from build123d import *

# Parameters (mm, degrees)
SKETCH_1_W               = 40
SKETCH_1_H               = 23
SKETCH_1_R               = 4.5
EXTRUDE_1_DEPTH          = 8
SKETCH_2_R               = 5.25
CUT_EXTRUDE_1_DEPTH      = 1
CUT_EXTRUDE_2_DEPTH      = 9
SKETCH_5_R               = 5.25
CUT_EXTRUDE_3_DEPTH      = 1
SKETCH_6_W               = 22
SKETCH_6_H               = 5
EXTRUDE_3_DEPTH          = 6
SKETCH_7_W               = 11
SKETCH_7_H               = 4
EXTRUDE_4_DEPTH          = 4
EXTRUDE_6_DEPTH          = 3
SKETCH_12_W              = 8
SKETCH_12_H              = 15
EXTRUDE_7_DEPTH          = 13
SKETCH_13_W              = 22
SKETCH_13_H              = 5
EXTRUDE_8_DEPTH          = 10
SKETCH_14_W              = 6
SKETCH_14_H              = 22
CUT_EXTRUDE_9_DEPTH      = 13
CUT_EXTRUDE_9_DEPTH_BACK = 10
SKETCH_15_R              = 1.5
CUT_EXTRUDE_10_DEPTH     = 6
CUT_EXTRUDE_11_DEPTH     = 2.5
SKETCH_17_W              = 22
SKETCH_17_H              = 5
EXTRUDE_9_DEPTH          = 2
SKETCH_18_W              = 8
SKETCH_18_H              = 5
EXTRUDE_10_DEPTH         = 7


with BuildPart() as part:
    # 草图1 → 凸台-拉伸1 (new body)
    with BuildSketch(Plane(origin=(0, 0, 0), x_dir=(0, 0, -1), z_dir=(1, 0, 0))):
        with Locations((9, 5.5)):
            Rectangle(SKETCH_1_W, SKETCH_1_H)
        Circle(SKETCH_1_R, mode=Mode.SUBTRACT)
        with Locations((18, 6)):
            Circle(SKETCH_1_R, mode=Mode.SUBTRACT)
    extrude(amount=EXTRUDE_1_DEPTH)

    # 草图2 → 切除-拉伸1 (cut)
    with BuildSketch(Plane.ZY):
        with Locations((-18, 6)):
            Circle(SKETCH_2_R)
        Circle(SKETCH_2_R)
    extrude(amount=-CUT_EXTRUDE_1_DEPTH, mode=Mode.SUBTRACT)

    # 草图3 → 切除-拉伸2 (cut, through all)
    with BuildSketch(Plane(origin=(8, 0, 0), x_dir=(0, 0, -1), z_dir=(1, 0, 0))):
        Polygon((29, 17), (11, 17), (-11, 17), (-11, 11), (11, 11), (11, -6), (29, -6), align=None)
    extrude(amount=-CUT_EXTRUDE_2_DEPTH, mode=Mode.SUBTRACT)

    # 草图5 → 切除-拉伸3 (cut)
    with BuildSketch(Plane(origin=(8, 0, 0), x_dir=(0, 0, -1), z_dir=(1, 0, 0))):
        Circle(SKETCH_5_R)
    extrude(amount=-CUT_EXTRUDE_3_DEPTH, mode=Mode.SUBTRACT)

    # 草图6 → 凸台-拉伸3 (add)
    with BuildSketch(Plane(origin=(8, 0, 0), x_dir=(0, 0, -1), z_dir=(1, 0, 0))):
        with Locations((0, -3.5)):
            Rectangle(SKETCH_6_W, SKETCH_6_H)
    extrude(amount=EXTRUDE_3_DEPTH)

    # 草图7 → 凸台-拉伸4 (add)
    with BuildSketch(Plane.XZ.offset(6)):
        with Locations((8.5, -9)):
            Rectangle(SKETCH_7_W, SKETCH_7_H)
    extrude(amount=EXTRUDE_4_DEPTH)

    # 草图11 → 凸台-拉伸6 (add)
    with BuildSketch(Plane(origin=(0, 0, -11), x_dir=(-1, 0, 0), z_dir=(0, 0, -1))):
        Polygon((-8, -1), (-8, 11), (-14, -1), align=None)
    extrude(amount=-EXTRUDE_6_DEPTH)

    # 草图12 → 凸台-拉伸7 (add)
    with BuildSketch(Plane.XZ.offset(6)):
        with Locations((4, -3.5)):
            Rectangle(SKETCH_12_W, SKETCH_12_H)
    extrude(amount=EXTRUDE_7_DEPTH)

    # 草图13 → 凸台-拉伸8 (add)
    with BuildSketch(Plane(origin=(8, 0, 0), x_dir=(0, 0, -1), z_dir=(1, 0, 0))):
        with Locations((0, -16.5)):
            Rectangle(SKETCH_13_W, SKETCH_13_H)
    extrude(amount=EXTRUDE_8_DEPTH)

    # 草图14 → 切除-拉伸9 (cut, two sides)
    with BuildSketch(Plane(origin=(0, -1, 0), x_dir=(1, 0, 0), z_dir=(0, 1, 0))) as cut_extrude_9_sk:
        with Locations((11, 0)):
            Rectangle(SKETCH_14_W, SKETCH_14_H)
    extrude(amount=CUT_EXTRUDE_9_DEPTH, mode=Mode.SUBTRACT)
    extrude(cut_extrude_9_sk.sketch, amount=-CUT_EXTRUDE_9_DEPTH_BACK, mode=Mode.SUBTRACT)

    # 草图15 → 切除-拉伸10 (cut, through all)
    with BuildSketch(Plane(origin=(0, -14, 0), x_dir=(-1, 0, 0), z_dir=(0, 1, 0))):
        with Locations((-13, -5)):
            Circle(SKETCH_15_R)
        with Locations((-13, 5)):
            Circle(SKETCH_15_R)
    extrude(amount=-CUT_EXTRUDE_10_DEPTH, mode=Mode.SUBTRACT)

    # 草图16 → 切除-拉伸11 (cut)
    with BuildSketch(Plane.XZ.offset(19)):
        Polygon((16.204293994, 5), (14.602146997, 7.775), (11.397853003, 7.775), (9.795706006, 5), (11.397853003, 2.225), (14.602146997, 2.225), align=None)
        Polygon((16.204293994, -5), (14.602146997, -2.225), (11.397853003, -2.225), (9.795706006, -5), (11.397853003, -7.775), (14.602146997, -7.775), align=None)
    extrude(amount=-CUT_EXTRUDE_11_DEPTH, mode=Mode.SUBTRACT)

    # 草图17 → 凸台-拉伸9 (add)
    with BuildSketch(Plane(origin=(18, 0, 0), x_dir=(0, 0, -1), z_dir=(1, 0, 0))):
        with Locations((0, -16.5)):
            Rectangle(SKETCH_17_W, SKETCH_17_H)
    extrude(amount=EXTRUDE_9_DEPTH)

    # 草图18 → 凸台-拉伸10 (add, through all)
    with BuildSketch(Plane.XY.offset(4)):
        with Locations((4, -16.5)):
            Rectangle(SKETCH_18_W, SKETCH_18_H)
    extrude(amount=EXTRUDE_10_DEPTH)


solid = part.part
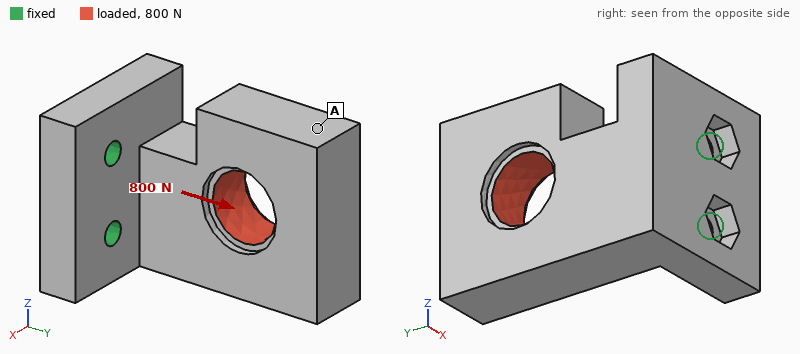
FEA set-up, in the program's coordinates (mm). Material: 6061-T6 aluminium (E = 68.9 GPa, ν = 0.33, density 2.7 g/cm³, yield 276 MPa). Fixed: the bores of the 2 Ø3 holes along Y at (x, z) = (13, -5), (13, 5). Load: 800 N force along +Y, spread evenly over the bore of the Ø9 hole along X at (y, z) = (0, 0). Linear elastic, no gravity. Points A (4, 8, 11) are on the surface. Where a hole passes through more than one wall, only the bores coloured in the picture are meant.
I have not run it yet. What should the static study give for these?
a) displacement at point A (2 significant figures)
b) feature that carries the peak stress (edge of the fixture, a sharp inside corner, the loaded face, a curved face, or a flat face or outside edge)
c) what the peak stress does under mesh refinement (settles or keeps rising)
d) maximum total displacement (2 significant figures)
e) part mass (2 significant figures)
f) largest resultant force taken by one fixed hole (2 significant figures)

0.13 mm
edge of the fixture
keeps rising
0.15 mm
15 g
410 N
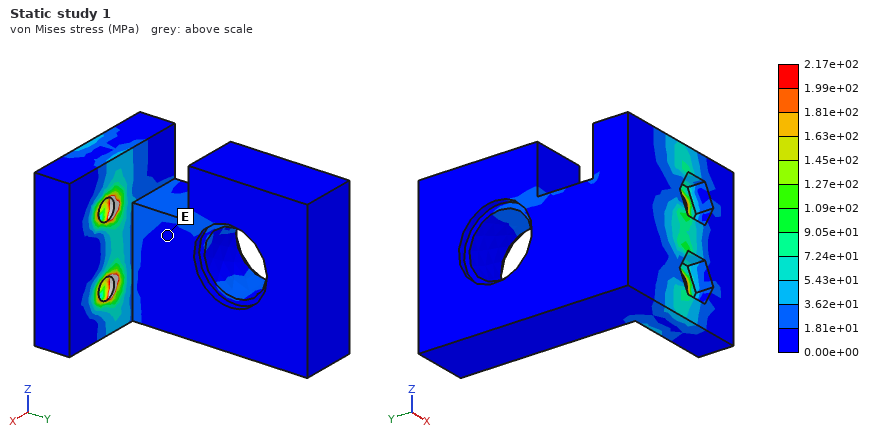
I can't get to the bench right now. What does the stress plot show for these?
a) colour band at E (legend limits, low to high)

0.00e+00 to 1.81e+01 MPa
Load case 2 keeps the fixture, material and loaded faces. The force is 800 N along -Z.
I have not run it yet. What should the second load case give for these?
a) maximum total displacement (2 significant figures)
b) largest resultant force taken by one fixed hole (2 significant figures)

0.14 mm
1.2 kN
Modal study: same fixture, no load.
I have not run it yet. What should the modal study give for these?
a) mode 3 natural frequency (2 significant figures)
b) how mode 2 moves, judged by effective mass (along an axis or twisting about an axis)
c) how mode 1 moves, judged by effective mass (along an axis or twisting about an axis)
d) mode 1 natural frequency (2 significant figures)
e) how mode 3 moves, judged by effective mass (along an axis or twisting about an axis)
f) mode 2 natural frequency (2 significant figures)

11 kHz
along Z
along X
2700 Hz
along Y
4800 Hz
